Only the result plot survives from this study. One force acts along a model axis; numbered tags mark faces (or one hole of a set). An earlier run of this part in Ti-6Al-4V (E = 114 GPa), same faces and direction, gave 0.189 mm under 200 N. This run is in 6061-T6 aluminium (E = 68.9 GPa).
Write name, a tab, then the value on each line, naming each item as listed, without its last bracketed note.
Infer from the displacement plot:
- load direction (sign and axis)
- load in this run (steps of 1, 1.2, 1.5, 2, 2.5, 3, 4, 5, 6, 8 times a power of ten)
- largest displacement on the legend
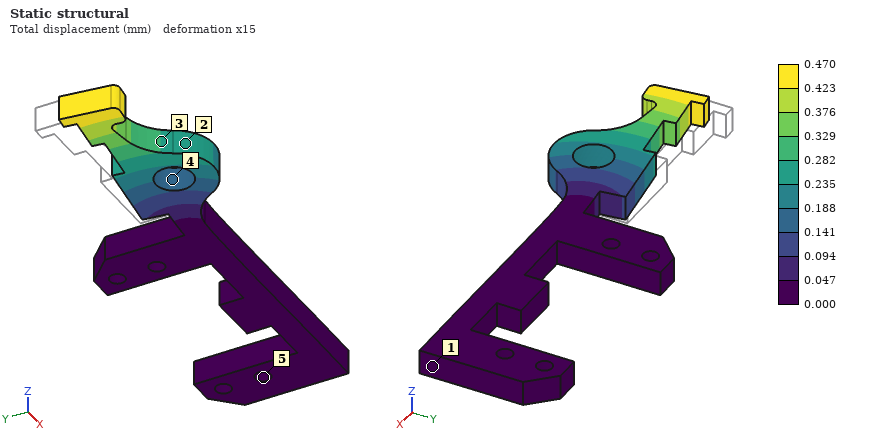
load direction	-Y
load in this run	300 N
largest displacement on the legend	0.470 mm
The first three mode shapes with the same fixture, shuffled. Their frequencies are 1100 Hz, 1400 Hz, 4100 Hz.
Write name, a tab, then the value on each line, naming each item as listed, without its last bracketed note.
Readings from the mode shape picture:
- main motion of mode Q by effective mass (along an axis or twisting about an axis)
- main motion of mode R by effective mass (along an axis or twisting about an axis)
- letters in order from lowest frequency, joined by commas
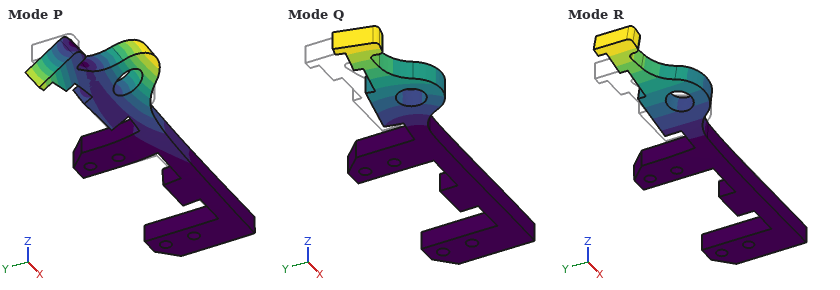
main motion of mode Q by effective mass	along Y
main motion of mode R by effective mass	along Z
letters in order from lowest frequency, joined by commas	R, Q, P
